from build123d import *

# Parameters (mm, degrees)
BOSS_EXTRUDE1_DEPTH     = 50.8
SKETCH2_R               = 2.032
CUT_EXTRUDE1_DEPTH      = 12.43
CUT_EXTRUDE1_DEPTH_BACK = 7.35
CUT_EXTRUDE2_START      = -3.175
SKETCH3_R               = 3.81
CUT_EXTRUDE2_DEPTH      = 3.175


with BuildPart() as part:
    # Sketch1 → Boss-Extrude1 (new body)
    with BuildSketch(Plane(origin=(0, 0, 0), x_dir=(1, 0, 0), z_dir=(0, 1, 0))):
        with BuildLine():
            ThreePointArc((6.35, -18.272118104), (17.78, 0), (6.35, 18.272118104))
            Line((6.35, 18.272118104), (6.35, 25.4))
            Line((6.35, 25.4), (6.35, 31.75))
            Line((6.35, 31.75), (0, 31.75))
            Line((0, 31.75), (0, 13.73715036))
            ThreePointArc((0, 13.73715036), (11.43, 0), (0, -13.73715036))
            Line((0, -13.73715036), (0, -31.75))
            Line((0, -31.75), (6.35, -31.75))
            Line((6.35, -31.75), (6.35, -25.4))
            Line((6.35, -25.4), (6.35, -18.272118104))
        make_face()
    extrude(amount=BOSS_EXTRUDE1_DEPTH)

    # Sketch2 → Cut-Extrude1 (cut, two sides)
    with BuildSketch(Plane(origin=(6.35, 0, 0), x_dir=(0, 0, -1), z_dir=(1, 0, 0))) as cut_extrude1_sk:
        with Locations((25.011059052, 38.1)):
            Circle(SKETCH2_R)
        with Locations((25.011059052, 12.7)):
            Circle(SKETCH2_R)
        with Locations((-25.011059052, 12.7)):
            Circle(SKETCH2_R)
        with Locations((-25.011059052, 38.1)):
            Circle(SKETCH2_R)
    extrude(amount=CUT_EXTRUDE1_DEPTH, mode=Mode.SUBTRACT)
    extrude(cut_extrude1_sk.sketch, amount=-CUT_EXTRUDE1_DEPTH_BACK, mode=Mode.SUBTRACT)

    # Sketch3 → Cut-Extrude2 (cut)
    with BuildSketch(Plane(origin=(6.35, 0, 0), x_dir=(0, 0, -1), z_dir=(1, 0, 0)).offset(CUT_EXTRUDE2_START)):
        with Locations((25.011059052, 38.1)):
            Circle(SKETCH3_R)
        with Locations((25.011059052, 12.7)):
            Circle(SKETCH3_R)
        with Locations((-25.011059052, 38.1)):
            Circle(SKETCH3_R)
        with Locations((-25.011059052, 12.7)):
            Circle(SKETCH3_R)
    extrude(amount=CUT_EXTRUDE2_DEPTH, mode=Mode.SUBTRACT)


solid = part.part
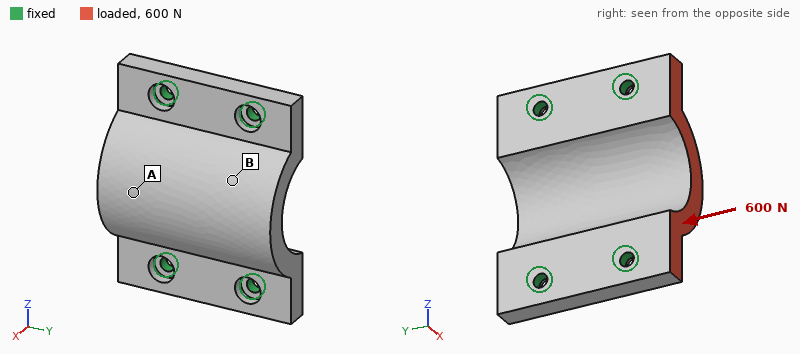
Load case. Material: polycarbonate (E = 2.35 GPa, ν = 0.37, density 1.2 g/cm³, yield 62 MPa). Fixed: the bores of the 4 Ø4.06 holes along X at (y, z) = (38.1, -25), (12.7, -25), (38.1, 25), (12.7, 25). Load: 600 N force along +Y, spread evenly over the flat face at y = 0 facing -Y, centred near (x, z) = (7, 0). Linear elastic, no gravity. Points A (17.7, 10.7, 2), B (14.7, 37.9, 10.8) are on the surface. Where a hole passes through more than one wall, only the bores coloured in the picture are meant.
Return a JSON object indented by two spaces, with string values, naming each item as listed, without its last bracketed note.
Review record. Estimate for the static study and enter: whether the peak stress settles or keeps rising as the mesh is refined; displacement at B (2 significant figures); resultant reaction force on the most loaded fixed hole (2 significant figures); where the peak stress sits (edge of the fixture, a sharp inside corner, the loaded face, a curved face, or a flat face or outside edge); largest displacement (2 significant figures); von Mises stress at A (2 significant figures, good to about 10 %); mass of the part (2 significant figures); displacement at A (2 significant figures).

{
  "whether the peak stress settles or keeps rising as the mesh is refined": "keeps rising",
  "displacement at B": "42 µm",
  "resultant reaction force on the most loaded fixed hole": "220 N",
  "where the peak stress sits": "edge of the fixture",
  "largest displacement": "87 µm",
  "von Mises stress at A": "1.6 MPa",
  "mass of the part": "28 g",
  "displacement at A": "65 µm"
}
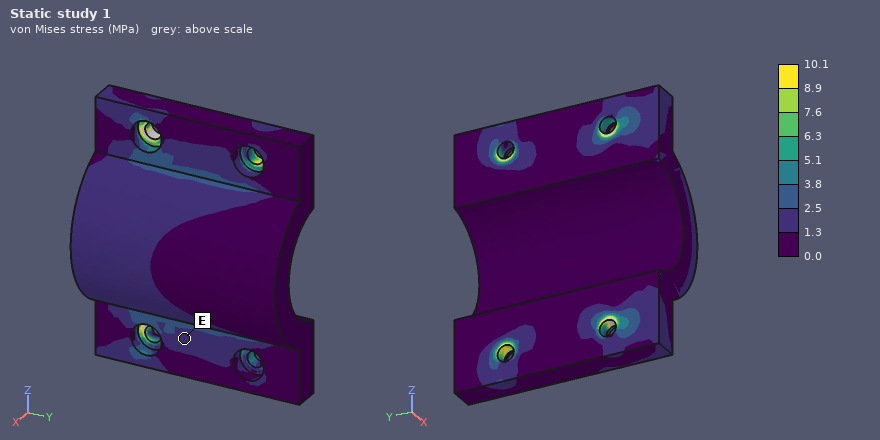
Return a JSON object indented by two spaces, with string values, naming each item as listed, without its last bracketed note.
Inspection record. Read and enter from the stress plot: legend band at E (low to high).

{
  "legend band at E": "1.3 to 2.5 MPa"
}
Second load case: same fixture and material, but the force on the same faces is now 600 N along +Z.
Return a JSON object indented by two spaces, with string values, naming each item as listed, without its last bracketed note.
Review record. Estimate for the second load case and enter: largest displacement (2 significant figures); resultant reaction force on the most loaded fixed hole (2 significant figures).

{
  "largest displacement": "0.13 mm",
  "resultant reaction force on the most loaded fixed hole": "300 N"
}
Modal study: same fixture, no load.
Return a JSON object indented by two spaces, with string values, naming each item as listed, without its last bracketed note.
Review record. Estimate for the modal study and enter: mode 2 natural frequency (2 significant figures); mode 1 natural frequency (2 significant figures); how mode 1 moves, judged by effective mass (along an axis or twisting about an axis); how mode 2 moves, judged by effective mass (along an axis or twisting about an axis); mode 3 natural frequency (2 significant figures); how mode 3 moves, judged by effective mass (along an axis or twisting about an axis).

{
  "mode 2 natural frequency": "3800 Hz",
  "mode 1 natural frequency": "2900 Hz",
  "how mode 1 moves, judged by effective mass": "along Y",
  "how mode 2 moves, judged by effective mass": "along X",
  "mode 3 natural frequency": "4600 Hz",
  "how mode 3 moves, judged by effective mass": "along Z"
}
